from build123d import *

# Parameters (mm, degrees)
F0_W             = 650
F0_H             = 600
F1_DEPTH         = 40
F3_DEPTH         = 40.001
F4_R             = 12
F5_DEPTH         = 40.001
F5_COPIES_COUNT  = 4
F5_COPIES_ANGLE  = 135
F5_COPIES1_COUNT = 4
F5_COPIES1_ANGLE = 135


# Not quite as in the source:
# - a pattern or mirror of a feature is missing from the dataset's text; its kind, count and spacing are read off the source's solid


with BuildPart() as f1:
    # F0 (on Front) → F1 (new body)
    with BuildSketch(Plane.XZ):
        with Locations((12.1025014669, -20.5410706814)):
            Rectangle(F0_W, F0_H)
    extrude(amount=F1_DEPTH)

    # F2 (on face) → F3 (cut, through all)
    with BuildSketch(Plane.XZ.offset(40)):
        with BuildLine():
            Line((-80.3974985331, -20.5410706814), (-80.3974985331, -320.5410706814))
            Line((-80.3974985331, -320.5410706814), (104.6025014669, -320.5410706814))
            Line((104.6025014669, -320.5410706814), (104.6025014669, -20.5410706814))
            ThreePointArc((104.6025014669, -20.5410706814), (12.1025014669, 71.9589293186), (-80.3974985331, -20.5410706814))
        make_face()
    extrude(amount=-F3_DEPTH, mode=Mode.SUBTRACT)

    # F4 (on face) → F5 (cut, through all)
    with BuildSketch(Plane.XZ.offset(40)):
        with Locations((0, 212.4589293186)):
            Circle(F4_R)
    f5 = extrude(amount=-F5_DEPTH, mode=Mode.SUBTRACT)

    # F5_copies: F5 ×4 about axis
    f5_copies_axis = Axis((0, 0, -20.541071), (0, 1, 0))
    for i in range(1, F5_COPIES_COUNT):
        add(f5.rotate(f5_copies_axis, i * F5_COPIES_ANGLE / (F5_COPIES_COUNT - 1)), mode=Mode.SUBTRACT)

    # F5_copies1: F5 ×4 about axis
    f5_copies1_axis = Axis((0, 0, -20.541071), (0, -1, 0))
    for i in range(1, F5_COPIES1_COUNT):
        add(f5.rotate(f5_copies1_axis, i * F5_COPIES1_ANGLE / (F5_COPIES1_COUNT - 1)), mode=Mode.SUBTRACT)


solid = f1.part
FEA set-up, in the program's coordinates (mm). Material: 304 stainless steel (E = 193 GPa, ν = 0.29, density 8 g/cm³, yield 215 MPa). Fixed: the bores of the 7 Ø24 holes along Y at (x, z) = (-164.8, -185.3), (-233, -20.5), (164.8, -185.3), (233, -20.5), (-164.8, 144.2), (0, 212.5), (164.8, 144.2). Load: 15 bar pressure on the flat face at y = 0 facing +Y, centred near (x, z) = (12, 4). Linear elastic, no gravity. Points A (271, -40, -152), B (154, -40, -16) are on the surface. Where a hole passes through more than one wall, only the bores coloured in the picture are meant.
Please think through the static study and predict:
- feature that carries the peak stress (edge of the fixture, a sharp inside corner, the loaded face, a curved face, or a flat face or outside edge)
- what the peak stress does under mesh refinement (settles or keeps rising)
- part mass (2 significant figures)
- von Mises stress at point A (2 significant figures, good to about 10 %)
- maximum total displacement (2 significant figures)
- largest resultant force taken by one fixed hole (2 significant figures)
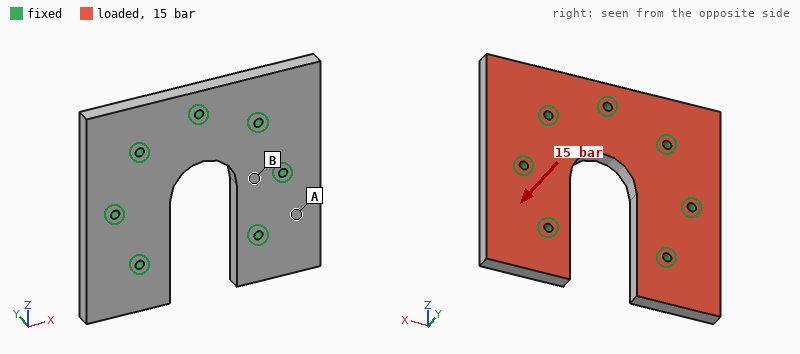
edge of the fixture
keeps rising
100 kg
25 MPa
0.28 mm
85 kN
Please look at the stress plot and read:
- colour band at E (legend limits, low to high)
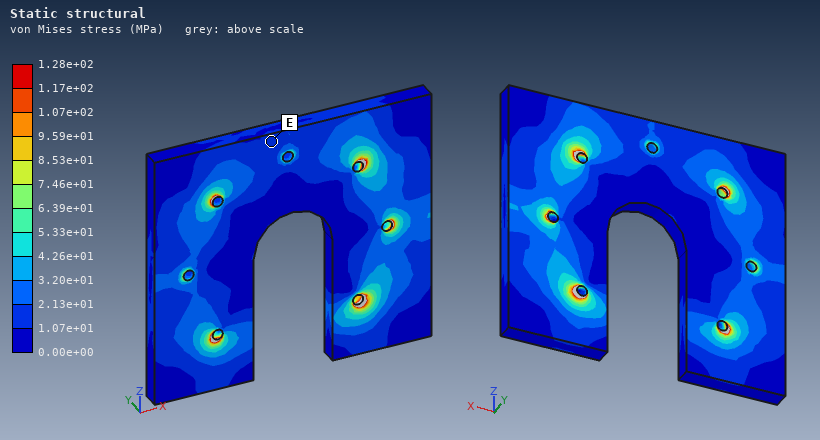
1.07e+01 to 2.13e+01 MPa
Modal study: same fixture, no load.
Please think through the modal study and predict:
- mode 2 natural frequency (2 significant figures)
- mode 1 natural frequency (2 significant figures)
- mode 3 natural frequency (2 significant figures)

960 Hz
910 Hz
1100 Hz
